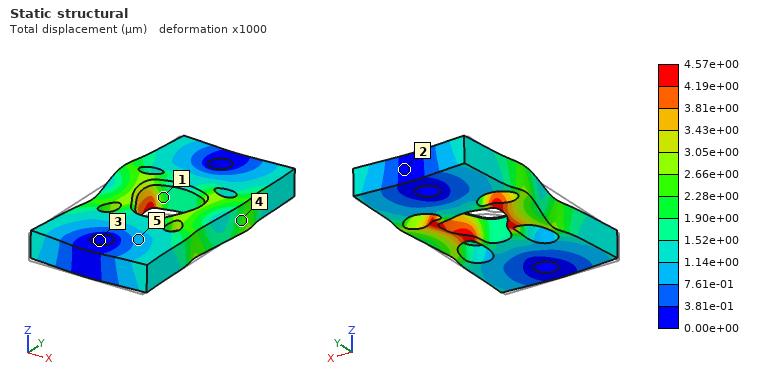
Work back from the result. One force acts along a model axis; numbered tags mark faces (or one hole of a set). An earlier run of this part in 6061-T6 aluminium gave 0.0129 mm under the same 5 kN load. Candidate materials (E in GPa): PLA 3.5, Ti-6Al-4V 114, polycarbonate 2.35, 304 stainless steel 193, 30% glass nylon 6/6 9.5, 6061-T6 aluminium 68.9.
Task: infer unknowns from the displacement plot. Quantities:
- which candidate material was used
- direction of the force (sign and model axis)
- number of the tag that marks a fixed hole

304 stainless steel
+Y
3
